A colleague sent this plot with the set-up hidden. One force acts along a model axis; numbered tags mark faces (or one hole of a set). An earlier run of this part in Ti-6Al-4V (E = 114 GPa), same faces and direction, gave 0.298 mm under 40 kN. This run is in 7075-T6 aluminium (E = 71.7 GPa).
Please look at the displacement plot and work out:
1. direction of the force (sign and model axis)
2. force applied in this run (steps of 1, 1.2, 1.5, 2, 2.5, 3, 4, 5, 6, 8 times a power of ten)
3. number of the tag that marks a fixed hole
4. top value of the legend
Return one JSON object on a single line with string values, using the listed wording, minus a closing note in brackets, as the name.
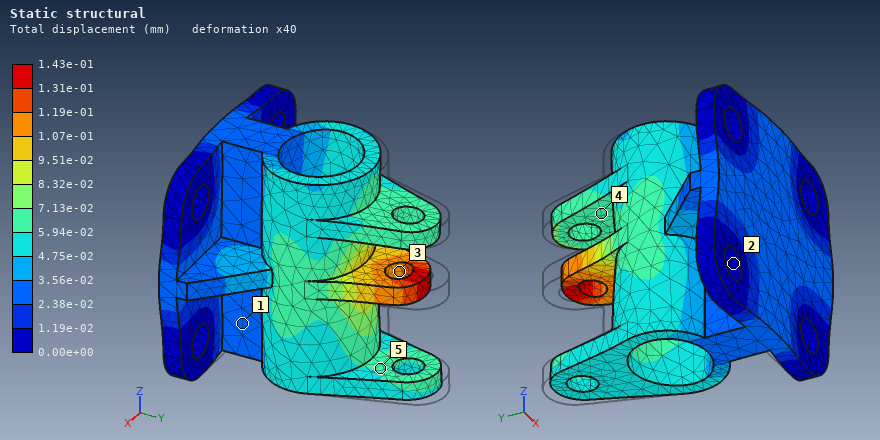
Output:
{"direction of the force": "-Y", "force applied in this run": "12 kN", "number of the tag that marks a fixed hole": "2", "top value of the legend": "1.43e-01 mm"}
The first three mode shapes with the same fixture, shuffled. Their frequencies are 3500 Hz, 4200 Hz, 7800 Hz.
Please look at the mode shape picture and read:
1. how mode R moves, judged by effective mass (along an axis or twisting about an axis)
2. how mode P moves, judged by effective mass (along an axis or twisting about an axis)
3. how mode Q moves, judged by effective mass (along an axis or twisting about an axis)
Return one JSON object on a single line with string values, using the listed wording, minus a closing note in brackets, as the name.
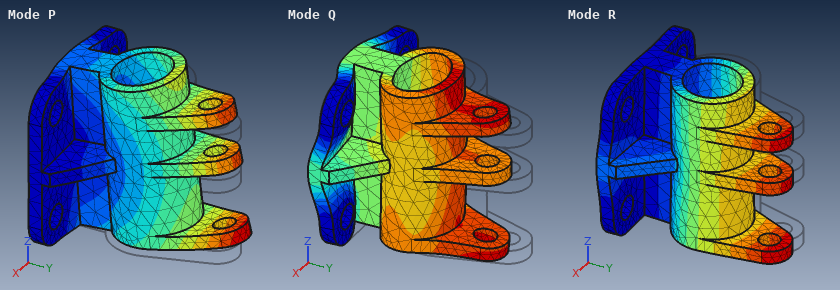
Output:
{"how mode R moves, judged by effective mass": "along X", "how mode P moves, judged by effective mass": "along Z", "how mode Q moves, judged by effective mass": "along Y"}
